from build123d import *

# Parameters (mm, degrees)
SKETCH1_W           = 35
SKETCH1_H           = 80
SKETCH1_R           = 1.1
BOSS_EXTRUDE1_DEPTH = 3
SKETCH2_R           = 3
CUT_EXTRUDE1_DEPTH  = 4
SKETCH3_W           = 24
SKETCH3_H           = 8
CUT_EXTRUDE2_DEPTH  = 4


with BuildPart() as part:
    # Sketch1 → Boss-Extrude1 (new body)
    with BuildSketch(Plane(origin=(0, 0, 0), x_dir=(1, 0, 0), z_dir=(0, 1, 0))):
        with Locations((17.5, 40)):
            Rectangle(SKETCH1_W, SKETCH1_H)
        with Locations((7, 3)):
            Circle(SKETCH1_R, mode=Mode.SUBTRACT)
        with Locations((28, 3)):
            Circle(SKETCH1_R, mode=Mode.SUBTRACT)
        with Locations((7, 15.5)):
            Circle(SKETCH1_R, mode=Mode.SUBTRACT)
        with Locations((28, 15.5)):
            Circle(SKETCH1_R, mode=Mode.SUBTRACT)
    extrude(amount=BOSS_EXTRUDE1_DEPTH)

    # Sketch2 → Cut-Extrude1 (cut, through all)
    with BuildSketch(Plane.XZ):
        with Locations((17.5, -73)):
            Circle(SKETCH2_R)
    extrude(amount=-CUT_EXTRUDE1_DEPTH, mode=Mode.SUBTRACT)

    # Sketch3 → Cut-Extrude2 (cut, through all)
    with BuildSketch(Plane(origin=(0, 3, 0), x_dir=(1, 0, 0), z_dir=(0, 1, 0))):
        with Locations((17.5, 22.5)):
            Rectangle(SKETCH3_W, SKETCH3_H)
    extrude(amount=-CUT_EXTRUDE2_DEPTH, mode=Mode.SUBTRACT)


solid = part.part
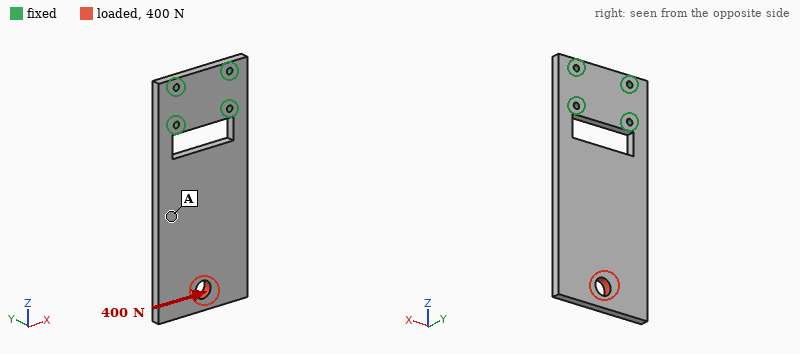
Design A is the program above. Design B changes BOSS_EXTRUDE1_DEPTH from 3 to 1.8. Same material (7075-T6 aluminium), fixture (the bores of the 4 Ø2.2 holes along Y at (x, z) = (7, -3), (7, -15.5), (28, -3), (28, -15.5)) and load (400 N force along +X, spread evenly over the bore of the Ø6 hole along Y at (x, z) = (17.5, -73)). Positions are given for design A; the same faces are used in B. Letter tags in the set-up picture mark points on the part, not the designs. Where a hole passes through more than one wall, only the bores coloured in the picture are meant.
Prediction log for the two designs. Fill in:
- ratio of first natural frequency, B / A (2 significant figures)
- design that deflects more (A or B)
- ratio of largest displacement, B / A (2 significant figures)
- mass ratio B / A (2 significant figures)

0.61
B
1.7
0.60
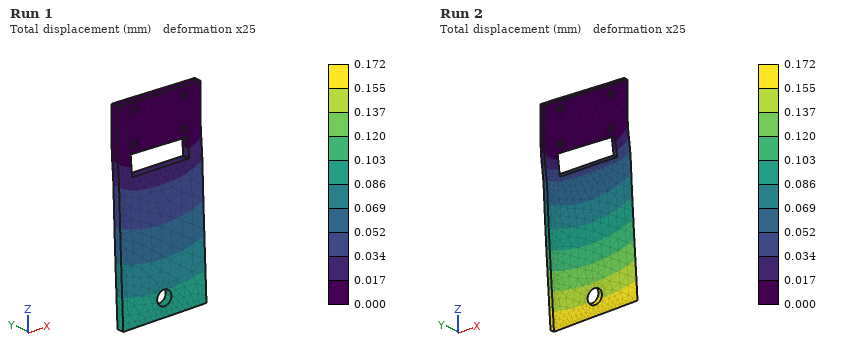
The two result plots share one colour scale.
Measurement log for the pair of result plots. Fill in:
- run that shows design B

Run 2
